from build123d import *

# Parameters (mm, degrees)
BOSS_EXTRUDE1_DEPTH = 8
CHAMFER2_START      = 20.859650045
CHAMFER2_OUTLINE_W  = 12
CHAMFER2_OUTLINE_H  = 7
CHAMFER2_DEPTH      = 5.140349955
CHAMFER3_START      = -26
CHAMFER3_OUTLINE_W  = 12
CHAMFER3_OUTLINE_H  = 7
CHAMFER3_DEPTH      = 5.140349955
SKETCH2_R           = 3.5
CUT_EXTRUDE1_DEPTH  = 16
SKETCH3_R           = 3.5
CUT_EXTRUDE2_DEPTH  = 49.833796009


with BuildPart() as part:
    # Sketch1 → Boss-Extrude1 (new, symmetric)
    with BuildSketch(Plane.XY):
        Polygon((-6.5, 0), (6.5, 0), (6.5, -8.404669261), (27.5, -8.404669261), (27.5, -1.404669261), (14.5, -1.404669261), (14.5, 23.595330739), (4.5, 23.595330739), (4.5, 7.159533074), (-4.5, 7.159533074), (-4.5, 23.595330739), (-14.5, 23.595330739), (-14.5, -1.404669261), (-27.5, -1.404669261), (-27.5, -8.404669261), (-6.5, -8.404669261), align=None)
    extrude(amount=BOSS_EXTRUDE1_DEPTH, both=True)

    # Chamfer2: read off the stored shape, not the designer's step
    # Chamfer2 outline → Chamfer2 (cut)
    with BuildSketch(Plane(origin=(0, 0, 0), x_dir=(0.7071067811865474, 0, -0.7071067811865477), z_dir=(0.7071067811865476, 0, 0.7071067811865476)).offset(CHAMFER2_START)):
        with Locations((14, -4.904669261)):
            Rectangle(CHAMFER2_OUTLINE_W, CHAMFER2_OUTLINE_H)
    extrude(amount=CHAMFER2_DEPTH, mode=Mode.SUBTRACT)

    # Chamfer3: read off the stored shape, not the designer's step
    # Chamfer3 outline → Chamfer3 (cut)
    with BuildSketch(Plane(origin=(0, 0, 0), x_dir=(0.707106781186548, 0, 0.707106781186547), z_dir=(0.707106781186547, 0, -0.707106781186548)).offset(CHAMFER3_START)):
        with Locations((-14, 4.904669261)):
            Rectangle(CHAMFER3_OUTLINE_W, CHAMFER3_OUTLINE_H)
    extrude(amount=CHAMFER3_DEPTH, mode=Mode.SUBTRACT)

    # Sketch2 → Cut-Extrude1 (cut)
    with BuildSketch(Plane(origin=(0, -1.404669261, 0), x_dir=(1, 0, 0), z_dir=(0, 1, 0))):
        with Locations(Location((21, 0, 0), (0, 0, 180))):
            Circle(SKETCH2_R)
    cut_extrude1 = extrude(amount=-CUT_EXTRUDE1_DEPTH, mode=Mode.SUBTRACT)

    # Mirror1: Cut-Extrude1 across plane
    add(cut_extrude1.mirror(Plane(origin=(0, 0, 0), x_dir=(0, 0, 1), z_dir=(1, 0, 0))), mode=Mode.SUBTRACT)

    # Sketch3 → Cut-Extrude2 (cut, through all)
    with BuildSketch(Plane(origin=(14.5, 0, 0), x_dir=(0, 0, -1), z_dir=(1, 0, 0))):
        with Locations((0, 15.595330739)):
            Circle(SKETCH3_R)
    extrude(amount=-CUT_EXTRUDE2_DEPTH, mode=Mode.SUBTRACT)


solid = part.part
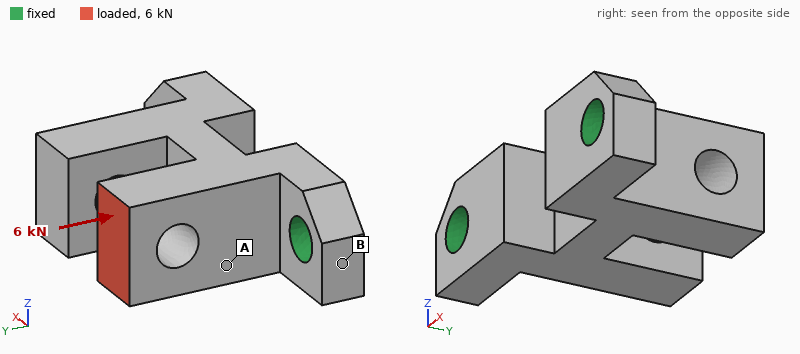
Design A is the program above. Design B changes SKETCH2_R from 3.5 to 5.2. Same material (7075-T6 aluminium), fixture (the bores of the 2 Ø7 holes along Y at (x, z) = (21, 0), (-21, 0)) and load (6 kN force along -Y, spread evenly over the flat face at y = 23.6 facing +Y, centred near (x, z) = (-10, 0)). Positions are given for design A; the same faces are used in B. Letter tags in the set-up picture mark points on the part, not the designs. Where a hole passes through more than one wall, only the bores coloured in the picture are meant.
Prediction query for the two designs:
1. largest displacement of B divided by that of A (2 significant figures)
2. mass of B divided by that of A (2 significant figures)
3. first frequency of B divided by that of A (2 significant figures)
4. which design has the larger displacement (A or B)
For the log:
0.81
0.95
1.2
A
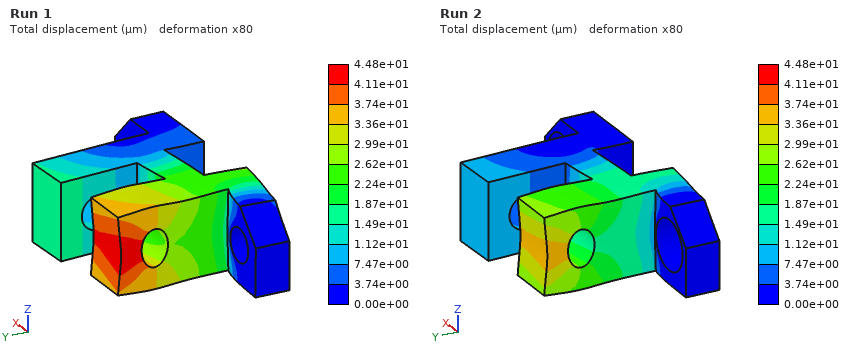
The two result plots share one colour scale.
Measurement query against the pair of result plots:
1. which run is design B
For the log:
Run 2
